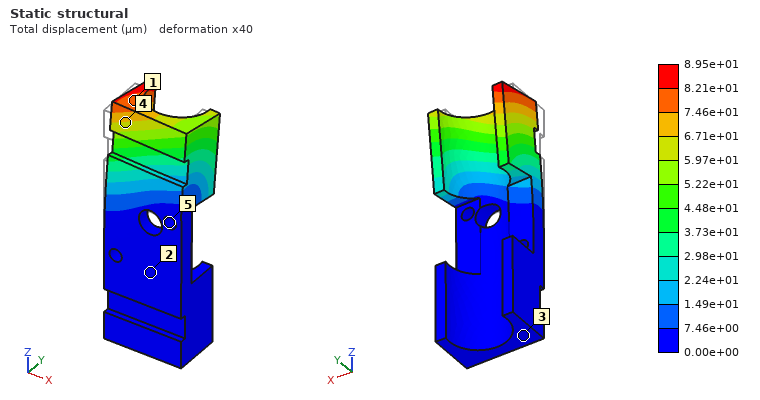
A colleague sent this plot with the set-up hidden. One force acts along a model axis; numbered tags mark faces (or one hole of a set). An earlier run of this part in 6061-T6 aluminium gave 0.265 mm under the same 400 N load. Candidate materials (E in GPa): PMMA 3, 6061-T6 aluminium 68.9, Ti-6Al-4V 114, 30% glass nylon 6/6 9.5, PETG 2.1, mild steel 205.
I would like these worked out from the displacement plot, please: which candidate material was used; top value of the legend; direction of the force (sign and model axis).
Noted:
mild steel
8.95e+01 µm
+Y
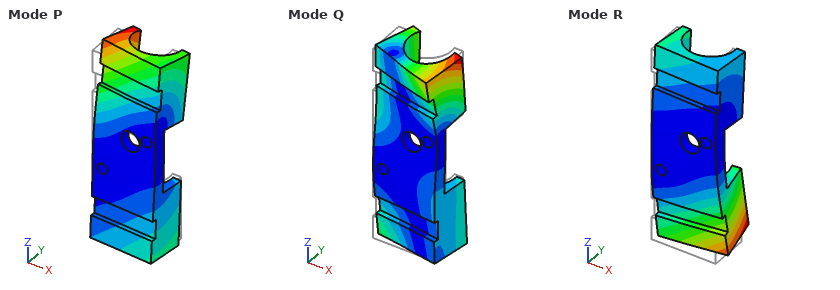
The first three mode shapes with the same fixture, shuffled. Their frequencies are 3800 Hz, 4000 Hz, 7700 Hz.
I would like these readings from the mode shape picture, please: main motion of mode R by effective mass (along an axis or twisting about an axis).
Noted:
along Y
